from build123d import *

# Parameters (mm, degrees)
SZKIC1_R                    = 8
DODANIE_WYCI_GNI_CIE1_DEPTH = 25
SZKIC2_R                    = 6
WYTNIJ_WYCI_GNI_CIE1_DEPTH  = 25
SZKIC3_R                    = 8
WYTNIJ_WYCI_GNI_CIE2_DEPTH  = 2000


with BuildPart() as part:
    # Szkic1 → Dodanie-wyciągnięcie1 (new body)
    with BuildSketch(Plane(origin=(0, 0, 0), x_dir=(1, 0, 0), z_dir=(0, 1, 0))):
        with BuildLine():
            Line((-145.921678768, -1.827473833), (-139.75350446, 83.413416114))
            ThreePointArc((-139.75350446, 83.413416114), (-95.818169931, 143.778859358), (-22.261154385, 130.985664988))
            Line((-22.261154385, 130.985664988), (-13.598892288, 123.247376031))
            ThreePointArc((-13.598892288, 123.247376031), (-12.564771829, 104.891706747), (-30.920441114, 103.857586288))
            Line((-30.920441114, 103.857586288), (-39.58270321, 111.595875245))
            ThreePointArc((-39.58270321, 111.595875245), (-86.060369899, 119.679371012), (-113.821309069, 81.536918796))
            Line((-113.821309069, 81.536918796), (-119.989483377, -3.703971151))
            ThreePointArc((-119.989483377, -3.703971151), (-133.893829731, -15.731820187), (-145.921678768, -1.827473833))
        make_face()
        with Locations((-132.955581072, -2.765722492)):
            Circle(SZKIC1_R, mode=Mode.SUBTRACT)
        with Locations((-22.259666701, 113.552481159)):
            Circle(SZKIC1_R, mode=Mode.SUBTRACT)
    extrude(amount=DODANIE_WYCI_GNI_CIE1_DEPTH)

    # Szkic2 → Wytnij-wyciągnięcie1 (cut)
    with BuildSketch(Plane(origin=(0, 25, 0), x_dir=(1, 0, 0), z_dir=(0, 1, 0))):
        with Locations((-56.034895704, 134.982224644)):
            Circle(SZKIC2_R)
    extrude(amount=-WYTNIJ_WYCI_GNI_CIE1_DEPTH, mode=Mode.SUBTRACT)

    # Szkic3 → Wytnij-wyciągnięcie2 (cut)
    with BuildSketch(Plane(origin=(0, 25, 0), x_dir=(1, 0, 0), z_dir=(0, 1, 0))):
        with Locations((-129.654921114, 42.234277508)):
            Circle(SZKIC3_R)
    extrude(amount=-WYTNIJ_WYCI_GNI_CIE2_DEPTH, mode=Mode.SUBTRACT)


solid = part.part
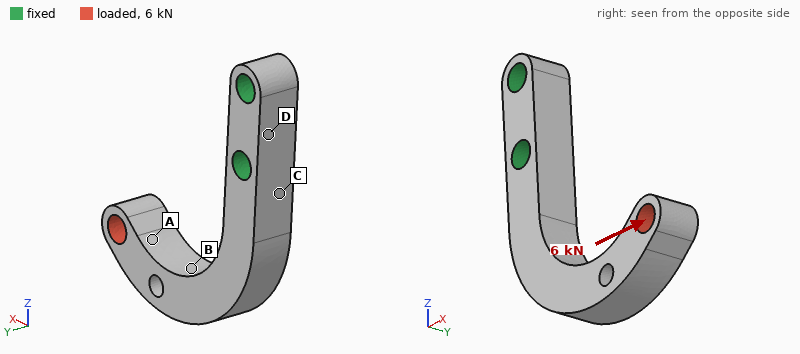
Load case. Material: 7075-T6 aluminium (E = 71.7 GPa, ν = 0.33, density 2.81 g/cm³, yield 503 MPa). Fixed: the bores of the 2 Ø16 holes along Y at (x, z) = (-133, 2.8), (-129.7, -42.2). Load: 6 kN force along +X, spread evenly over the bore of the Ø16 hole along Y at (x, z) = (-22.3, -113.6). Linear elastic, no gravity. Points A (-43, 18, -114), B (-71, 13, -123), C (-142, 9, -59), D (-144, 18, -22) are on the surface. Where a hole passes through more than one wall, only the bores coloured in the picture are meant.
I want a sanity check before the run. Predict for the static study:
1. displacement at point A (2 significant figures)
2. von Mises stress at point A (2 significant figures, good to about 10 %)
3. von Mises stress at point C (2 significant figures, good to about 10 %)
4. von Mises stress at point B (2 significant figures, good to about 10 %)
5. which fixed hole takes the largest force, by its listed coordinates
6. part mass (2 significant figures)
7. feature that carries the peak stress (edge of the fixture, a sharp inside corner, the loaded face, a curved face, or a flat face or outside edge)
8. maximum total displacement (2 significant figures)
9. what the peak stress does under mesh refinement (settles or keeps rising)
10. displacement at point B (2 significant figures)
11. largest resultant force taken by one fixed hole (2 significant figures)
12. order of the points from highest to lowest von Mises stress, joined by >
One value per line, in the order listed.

0.53 mm
45 MPa
120 MPa
71 MPa
(-129.7, -42.2)
400 g
edge of the fixture
0.59 mm
keeps rising
0.47 mm
6.7 kN
C > B > A > D
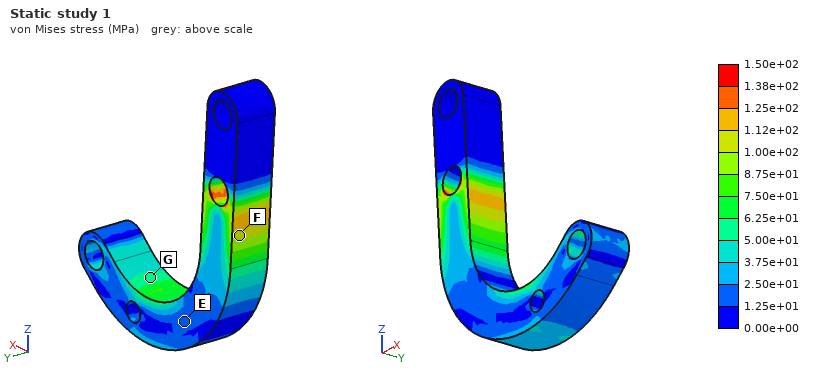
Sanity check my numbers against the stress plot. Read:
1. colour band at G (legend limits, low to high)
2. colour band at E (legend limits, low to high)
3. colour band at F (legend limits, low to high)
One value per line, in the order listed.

5.00e+01 to 6.25e+01 MPa
1.25e+01 to 2.50e+01 MPa
1.00e+02 to 1.12e+02 MPa
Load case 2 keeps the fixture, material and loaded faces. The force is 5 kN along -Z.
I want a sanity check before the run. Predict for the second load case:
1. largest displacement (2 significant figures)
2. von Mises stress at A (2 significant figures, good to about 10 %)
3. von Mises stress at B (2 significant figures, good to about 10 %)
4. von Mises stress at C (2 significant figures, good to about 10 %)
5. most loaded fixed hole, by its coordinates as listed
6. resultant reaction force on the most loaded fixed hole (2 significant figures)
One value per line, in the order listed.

2.5 mm
20 MPa
110 MPa
180 MPa
(-129.7, -42.2)
5.1 kN
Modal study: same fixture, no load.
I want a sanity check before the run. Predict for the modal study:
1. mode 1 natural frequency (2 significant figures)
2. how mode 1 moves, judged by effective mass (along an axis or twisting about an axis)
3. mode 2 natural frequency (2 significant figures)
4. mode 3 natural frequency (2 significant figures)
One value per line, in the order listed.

700 Hz
along Y
770 Hz
2000 Hz
